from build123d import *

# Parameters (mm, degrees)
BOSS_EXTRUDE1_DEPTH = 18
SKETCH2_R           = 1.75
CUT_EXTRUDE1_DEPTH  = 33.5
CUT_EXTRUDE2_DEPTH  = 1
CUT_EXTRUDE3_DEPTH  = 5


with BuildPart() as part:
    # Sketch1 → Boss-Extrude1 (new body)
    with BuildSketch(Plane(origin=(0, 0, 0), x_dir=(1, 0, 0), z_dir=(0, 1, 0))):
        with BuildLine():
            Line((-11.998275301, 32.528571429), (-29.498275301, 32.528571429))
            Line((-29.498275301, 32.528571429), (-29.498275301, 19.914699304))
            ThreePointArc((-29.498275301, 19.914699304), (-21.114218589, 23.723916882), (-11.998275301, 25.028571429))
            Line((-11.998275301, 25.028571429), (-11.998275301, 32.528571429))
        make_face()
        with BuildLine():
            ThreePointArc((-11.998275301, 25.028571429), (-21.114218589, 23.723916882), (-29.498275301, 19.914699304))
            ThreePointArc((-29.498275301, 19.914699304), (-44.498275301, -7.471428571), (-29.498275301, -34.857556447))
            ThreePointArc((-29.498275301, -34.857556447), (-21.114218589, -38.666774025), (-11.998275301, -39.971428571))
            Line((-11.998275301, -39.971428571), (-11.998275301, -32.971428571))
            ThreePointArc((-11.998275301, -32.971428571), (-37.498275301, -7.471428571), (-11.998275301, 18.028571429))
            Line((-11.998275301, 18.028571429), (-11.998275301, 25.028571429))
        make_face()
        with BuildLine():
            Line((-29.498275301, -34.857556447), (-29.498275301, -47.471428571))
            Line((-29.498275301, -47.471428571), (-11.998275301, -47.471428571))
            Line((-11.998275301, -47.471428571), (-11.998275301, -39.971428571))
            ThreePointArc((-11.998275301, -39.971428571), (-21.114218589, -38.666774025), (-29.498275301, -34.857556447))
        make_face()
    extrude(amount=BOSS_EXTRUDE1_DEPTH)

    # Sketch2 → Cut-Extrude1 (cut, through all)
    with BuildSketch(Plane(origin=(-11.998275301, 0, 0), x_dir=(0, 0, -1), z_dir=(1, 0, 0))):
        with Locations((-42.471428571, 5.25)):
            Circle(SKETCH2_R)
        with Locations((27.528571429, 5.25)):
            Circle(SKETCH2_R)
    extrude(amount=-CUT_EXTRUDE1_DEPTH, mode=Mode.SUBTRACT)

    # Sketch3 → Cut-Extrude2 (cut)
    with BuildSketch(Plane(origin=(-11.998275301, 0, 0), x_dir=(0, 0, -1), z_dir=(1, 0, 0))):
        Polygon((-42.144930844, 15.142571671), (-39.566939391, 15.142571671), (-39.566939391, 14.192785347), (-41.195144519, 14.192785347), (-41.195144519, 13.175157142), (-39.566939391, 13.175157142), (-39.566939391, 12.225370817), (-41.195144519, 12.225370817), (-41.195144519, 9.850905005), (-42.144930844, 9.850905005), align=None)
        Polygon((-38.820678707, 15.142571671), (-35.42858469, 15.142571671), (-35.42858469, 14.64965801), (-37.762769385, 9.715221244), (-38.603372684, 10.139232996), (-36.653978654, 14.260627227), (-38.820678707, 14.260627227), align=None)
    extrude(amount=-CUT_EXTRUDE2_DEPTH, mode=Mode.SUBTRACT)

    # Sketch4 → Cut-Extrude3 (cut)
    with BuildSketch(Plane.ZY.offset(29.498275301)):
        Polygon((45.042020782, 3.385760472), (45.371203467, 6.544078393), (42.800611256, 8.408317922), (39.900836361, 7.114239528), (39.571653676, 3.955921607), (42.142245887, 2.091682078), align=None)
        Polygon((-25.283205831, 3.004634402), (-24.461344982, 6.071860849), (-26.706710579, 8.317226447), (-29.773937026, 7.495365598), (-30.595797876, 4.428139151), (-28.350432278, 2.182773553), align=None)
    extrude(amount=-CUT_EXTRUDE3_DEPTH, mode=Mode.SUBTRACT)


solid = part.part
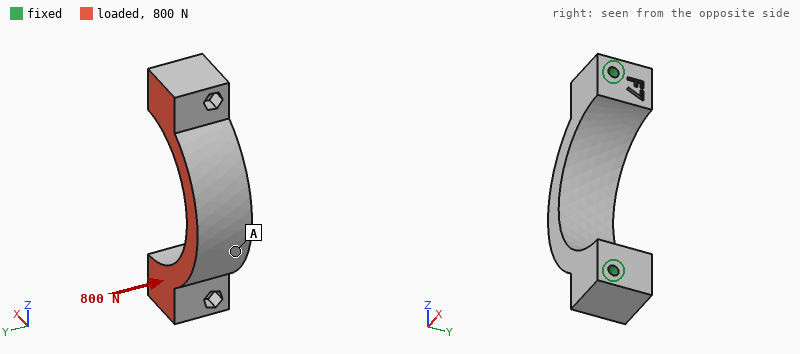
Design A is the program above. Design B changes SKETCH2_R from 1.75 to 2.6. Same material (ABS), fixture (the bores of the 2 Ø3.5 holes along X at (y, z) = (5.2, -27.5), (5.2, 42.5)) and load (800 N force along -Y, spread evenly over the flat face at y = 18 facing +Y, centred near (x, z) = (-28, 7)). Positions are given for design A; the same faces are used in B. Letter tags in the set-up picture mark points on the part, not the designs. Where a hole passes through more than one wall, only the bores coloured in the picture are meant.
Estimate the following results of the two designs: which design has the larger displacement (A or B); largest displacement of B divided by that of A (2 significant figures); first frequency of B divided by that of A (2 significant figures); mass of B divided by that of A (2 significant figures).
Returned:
A
0.74
1.2
0.98
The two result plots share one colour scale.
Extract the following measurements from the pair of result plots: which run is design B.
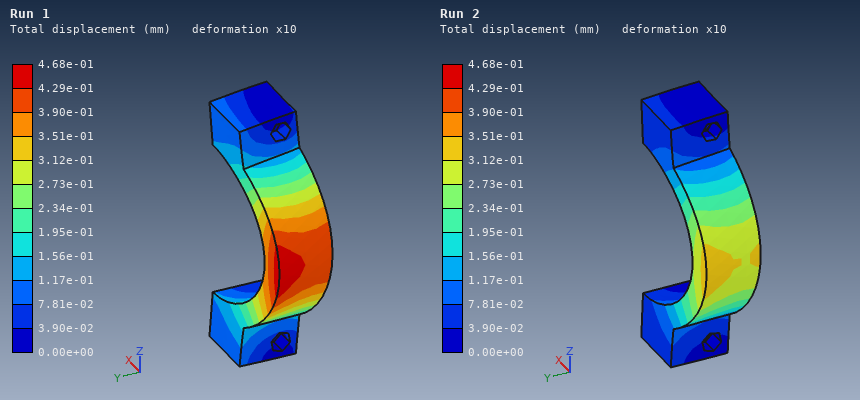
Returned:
Run 2
